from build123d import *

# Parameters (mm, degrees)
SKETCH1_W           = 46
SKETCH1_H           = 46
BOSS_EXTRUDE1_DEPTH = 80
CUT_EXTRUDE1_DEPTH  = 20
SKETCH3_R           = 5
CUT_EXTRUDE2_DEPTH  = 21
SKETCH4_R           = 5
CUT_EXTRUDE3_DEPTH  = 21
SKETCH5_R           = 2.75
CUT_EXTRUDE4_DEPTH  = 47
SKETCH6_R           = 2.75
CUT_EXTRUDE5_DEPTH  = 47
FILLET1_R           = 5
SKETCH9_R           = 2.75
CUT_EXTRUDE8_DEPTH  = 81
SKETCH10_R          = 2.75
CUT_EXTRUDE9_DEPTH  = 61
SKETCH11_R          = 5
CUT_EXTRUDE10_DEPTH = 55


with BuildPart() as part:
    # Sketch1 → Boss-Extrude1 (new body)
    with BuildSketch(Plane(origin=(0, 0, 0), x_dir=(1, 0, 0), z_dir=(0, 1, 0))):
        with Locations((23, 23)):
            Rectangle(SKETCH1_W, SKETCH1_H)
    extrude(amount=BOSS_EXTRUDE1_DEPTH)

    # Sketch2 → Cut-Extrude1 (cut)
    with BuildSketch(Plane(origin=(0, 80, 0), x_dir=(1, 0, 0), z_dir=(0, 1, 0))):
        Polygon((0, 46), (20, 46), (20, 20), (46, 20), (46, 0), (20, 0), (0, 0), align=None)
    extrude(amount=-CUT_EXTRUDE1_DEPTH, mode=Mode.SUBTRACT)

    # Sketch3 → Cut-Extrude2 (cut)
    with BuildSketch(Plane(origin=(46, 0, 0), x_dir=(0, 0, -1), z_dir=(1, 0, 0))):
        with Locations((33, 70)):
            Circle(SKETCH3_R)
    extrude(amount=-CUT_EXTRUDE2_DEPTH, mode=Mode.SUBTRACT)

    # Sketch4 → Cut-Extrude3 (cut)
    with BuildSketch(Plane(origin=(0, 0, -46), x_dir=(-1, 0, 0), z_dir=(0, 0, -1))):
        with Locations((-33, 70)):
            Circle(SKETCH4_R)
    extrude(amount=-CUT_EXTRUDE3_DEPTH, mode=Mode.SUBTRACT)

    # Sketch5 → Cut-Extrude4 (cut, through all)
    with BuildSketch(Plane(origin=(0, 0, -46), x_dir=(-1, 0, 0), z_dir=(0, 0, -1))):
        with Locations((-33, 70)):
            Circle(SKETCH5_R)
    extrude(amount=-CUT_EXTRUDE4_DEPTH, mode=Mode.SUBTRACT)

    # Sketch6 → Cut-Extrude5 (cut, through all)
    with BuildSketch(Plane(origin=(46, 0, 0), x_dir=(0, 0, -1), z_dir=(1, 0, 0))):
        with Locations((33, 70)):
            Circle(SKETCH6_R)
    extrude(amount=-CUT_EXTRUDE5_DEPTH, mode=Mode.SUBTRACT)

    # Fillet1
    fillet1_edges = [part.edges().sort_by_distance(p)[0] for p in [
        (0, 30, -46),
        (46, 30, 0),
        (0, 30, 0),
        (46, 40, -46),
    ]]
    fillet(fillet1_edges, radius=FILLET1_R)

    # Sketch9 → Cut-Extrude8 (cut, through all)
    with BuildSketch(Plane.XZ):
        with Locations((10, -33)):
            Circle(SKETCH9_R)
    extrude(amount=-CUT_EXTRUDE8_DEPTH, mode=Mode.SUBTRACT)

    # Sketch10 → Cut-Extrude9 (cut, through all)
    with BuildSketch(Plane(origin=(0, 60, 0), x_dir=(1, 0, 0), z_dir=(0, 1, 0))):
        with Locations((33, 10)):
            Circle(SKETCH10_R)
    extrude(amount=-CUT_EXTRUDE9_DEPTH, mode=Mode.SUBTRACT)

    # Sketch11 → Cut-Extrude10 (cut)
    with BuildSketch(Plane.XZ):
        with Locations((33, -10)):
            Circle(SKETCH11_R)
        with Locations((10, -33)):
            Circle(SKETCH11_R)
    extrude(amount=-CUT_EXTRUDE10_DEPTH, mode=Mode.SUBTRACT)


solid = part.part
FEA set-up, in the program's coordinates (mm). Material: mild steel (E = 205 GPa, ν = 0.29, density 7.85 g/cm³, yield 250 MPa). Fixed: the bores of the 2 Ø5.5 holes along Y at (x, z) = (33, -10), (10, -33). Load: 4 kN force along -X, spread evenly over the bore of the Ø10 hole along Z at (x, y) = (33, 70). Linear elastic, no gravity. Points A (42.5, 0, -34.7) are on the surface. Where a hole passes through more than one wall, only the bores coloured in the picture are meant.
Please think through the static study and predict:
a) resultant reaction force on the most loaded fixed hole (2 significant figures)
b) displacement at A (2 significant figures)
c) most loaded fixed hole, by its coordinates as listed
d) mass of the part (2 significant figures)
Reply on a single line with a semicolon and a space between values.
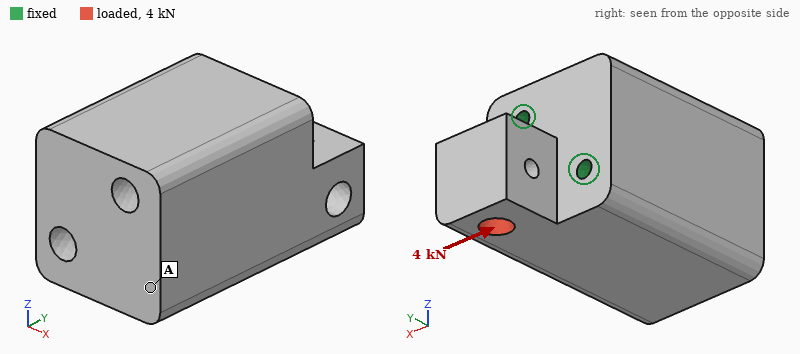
4.1 kN; 40 µm; (10, -33); 1000 g
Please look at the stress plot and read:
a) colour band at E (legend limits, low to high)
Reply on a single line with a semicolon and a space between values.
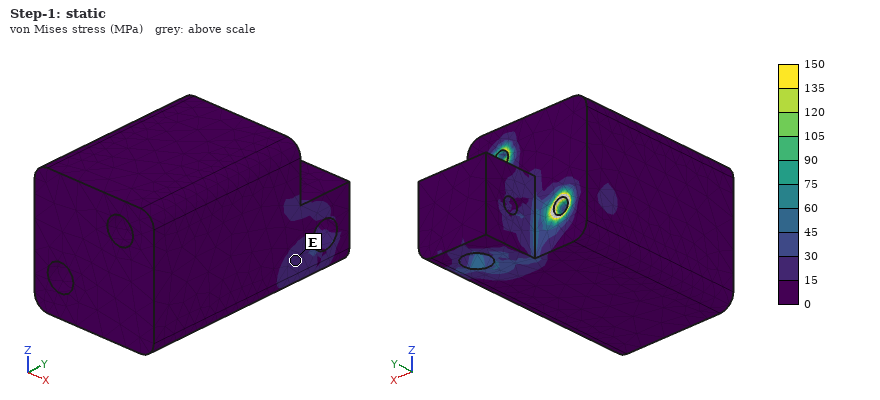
15 to 30 MPa
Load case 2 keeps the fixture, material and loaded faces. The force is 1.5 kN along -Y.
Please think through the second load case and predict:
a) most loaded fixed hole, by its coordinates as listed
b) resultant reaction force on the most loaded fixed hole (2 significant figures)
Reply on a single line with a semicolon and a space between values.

(10, -33); 1000 N
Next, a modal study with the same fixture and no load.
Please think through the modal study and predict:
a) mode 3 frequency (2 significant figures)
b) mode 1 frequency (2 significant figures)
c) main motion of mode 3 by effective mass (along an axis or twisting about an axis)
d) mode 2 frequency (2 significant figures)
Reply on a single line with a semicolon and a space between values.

8000 Hz; 1100 Hz; twisting about Y; 3900 Hz
